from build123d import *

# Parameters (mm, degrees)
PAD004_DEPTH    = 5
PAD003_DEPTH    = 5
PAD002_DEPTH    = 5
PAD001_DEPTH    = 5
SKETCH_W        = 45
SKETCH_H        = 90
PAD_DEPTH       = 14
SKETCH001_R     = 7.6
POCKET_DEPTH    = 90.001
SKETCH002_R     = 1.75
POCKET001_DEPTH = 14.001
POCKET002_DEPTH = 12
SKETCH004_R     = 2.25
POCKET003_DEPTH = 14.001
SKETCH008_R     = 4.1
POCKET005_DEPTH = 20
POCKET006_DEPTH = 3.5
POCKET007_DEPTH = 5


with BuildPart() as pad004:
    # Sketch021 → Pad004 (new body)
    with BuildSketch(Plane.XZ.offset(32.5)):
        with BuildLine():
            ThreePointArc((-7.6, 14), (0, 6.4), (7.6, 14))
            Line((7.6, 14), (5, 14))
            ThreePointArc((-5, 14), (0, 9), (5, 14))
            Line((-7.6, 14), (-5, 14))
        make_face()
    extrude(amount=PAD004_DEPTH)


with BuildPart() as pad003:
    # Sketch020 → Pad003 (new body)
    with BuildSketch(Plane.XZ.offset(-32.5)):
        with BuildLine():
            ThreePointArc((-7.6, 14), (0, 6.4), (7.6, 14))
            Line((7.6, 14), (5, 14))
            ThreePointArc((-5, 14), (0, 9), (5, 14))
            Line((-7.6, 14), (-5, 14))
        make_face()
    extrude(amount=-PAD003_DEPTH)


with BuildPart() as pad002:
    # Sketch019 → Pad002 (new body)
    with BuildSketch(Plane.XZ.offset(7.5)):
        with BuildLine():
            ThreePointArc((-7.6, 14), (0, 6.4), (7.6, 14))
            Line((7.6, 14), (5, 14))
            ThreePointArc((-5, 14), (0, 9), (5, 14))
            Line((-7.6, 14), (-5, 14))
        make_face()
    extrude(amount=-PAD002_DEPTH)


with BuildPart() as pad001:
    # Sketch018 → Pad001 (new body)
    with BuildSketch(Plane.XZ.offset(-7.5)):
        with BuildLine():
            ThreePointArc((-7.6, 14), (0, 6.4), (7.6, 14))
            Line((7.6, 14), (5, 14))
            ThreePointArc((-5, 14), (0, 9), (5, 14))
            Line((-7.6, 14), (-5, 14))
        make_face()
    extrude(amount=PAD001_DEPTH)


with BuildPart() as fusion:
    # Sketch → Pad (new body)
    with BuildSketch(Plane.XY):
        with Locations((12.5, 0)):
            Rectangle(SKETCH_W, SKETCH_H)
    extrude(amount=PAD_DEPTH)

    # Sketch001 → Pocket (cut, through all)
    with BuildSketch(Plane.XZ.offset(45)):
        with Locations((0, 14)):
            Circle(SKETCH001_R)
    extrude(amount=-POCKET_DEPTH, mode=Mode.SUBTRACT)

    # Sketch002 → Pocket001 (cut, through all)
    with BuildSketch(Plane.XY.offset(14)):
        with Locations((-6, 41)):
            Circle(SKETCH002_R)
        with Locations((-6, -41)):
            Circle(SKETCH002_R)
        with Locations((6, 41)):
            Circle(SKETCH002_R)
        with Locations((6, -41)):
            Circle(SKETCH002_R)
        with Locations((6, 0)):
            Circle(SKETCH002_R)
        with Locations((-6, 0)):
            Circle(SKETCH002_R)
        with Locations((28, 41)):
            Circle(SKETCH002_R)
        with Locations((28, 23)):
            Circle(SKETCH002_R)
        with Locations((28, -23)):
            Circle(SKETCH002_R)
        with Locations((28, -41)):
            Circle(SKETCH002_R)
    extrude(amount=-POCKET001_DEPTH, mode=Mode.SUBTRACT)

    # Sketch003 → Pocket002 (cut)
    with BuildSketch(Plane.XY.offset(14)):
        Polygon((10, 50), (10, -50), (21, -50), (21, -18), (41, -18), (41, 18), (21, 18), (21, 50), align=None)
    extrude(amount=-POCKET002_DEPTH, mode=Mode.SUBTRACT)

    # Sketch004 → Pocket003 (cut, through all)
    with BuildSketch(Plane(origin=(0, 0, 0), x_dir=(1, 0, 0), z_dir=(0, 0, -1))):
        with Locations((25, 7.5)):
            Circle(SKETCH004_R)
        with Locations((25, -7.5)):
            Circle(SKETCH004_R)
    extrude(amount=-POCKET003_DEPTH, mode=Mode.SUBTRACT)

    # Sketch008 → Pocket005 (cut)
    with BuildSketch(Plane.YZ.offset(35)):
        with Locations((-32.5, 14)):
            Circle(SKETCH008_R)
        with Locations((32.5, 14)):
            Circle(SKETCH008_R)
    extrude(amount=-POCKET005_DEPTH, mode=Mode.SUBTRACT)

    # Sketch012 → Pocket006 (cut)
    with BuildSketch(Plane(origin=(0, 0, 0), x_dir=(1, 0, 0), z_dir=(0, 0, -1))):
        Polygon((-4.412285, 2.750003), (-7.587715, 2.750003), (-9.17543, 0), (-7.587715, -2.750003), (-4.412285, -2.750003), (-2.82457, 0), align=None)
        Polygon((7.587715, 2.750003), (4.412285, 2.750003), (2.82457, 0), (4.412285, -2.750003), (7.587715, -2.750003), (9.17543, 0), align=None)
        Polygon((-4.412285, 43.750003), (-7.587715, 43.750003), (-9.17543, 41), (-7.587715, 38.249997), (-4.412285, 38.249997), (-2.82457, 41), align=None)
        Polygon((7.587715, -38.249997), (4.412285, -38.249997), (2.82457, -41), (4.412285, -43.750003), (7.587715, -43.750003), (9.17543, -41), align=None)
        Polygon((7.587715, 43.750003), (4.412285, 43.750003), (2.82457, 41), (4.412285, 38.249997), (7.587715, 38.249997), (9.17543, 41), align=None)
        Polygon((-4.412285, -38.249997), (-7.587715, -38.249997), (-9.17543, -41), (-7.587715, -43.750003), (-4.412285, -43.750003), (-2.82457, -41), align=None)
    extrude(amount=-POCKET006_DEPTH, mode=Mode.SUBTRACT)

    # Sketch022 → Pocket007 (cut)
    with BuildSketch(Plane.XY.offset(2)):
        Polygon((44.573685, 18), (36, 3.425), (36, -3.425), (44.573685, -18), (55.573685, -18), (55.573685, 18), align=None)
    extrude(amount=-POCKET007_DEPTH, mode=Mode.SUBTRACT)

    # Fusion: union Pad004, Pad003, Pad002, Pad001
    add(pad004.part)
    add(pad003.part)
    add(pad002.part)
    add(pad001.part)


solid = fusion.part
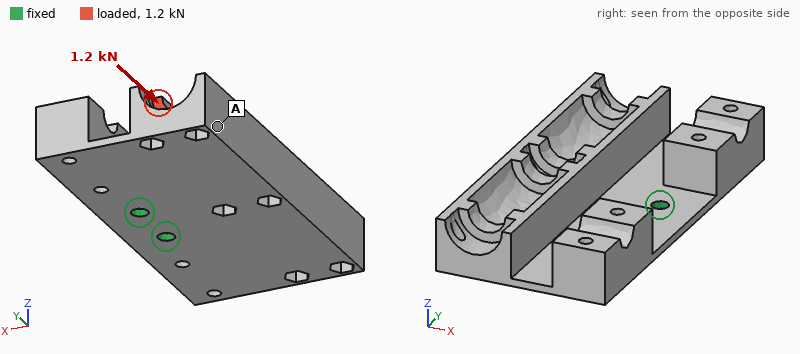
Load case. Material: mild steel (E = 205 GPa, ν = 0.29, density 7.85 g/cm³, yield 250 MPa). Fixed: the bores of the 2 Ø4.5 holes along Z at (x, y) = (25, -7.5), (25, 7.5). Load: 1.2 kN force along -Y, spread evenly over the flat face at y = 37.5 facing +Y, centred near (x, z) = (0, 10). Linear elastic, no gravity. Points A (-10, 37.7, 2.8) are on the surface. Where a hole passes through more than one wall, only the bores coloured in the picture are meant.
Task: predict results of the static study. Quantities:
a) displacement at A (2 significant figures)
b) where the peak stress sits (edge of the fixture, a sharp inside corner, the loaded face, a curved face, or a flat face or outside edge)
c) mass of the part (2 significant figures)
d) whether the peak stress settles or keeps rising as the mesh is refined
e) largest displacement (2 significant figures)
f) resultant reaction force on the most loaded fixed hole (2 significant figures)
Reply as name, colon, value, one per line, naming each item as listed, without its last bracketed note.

displacement at A: 0.15 mm
where the peak stress sits: edge of the fixture
mass of the part: 230 g
whether the peak stress settles or keeps rising as the mesh is refined: keeps rising
largest displacement: 0.20 mm
resultant reaction force on the most loaded fixed hole: 1.7 kN
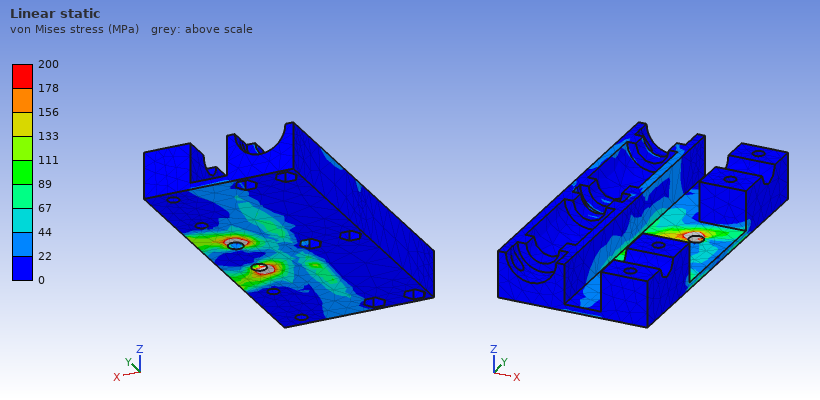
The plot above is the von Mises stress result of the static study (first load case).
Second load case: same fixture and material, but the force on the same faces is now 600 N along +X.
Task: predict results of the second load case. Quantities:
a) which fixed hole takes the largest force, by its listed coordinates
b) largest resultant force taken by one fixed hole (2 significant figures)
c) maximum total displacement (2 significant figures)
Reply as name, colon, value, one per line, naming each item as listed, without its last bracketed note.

which fixed hole takes the largest force, by its listed coordinates: (25, 7.5)
largest resultant force taken by one fixed hole: 1.5 kN
maximum total displacement: 0.26 mm
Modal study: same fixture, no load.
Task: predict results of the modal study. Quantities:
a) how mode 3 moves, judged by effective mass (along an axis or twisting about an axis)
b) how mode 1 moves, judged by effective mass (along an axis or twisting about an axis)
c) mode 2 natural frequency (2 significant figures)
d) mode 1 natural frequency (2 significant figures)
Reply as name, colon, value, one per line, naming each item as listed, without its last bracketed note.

how mode 3 moves, judged by effective mass: along Z
how mode 1 moves, judged by effective mass: along Z
mode 2 natural frequency: 680 Hz
mode 1 natural frequency: 560 Hz
